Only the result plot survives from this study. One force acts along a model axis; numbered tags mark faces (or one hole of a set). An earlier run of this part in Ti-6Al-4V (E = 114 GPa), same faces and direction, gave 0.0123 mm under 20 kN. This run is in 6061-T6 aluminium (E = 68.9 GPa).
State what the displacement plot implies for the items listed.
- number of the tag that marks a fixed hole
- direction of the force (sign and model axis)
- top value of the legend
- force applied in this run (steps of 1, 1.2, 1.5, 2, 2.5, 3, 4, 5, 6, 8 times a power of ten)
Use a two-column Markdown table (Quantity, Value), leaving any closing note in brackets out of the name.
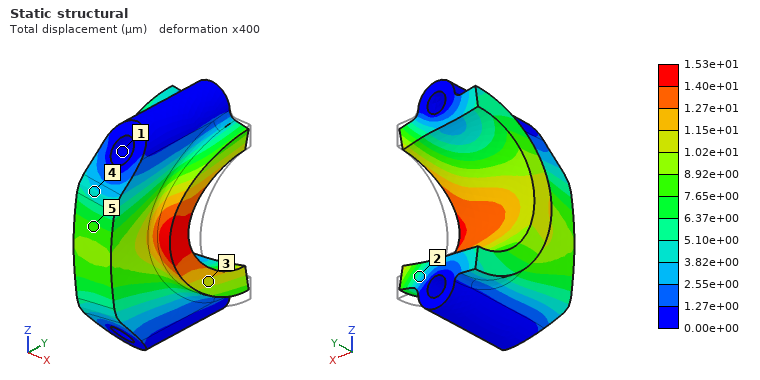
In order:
| Quantity | Value |
|---|---|
| number of the tag that marks a fixed hole | 1 |
| direction of the force | -X |
| top value of the legend | 1.53e+01 µm |
| force applied in this run | 15 kN |
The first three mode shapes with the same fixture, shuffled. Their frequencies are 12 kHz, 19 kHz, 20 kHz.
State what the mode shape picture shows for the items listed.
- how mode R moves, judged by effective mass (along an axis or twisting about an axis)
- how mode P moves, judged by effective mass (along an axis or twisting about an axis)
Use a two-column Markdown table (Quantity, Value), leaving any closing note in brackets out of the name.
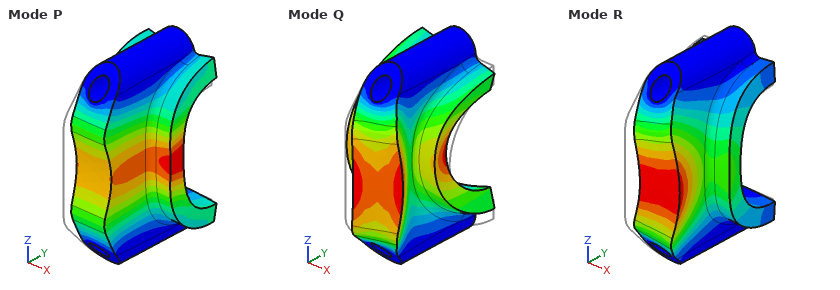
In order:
| Quantity | Value |
|---|---|
| how mode R moves, judged by effective mass | along X |
| how mode P moves, judged by effective mass | along Y |
